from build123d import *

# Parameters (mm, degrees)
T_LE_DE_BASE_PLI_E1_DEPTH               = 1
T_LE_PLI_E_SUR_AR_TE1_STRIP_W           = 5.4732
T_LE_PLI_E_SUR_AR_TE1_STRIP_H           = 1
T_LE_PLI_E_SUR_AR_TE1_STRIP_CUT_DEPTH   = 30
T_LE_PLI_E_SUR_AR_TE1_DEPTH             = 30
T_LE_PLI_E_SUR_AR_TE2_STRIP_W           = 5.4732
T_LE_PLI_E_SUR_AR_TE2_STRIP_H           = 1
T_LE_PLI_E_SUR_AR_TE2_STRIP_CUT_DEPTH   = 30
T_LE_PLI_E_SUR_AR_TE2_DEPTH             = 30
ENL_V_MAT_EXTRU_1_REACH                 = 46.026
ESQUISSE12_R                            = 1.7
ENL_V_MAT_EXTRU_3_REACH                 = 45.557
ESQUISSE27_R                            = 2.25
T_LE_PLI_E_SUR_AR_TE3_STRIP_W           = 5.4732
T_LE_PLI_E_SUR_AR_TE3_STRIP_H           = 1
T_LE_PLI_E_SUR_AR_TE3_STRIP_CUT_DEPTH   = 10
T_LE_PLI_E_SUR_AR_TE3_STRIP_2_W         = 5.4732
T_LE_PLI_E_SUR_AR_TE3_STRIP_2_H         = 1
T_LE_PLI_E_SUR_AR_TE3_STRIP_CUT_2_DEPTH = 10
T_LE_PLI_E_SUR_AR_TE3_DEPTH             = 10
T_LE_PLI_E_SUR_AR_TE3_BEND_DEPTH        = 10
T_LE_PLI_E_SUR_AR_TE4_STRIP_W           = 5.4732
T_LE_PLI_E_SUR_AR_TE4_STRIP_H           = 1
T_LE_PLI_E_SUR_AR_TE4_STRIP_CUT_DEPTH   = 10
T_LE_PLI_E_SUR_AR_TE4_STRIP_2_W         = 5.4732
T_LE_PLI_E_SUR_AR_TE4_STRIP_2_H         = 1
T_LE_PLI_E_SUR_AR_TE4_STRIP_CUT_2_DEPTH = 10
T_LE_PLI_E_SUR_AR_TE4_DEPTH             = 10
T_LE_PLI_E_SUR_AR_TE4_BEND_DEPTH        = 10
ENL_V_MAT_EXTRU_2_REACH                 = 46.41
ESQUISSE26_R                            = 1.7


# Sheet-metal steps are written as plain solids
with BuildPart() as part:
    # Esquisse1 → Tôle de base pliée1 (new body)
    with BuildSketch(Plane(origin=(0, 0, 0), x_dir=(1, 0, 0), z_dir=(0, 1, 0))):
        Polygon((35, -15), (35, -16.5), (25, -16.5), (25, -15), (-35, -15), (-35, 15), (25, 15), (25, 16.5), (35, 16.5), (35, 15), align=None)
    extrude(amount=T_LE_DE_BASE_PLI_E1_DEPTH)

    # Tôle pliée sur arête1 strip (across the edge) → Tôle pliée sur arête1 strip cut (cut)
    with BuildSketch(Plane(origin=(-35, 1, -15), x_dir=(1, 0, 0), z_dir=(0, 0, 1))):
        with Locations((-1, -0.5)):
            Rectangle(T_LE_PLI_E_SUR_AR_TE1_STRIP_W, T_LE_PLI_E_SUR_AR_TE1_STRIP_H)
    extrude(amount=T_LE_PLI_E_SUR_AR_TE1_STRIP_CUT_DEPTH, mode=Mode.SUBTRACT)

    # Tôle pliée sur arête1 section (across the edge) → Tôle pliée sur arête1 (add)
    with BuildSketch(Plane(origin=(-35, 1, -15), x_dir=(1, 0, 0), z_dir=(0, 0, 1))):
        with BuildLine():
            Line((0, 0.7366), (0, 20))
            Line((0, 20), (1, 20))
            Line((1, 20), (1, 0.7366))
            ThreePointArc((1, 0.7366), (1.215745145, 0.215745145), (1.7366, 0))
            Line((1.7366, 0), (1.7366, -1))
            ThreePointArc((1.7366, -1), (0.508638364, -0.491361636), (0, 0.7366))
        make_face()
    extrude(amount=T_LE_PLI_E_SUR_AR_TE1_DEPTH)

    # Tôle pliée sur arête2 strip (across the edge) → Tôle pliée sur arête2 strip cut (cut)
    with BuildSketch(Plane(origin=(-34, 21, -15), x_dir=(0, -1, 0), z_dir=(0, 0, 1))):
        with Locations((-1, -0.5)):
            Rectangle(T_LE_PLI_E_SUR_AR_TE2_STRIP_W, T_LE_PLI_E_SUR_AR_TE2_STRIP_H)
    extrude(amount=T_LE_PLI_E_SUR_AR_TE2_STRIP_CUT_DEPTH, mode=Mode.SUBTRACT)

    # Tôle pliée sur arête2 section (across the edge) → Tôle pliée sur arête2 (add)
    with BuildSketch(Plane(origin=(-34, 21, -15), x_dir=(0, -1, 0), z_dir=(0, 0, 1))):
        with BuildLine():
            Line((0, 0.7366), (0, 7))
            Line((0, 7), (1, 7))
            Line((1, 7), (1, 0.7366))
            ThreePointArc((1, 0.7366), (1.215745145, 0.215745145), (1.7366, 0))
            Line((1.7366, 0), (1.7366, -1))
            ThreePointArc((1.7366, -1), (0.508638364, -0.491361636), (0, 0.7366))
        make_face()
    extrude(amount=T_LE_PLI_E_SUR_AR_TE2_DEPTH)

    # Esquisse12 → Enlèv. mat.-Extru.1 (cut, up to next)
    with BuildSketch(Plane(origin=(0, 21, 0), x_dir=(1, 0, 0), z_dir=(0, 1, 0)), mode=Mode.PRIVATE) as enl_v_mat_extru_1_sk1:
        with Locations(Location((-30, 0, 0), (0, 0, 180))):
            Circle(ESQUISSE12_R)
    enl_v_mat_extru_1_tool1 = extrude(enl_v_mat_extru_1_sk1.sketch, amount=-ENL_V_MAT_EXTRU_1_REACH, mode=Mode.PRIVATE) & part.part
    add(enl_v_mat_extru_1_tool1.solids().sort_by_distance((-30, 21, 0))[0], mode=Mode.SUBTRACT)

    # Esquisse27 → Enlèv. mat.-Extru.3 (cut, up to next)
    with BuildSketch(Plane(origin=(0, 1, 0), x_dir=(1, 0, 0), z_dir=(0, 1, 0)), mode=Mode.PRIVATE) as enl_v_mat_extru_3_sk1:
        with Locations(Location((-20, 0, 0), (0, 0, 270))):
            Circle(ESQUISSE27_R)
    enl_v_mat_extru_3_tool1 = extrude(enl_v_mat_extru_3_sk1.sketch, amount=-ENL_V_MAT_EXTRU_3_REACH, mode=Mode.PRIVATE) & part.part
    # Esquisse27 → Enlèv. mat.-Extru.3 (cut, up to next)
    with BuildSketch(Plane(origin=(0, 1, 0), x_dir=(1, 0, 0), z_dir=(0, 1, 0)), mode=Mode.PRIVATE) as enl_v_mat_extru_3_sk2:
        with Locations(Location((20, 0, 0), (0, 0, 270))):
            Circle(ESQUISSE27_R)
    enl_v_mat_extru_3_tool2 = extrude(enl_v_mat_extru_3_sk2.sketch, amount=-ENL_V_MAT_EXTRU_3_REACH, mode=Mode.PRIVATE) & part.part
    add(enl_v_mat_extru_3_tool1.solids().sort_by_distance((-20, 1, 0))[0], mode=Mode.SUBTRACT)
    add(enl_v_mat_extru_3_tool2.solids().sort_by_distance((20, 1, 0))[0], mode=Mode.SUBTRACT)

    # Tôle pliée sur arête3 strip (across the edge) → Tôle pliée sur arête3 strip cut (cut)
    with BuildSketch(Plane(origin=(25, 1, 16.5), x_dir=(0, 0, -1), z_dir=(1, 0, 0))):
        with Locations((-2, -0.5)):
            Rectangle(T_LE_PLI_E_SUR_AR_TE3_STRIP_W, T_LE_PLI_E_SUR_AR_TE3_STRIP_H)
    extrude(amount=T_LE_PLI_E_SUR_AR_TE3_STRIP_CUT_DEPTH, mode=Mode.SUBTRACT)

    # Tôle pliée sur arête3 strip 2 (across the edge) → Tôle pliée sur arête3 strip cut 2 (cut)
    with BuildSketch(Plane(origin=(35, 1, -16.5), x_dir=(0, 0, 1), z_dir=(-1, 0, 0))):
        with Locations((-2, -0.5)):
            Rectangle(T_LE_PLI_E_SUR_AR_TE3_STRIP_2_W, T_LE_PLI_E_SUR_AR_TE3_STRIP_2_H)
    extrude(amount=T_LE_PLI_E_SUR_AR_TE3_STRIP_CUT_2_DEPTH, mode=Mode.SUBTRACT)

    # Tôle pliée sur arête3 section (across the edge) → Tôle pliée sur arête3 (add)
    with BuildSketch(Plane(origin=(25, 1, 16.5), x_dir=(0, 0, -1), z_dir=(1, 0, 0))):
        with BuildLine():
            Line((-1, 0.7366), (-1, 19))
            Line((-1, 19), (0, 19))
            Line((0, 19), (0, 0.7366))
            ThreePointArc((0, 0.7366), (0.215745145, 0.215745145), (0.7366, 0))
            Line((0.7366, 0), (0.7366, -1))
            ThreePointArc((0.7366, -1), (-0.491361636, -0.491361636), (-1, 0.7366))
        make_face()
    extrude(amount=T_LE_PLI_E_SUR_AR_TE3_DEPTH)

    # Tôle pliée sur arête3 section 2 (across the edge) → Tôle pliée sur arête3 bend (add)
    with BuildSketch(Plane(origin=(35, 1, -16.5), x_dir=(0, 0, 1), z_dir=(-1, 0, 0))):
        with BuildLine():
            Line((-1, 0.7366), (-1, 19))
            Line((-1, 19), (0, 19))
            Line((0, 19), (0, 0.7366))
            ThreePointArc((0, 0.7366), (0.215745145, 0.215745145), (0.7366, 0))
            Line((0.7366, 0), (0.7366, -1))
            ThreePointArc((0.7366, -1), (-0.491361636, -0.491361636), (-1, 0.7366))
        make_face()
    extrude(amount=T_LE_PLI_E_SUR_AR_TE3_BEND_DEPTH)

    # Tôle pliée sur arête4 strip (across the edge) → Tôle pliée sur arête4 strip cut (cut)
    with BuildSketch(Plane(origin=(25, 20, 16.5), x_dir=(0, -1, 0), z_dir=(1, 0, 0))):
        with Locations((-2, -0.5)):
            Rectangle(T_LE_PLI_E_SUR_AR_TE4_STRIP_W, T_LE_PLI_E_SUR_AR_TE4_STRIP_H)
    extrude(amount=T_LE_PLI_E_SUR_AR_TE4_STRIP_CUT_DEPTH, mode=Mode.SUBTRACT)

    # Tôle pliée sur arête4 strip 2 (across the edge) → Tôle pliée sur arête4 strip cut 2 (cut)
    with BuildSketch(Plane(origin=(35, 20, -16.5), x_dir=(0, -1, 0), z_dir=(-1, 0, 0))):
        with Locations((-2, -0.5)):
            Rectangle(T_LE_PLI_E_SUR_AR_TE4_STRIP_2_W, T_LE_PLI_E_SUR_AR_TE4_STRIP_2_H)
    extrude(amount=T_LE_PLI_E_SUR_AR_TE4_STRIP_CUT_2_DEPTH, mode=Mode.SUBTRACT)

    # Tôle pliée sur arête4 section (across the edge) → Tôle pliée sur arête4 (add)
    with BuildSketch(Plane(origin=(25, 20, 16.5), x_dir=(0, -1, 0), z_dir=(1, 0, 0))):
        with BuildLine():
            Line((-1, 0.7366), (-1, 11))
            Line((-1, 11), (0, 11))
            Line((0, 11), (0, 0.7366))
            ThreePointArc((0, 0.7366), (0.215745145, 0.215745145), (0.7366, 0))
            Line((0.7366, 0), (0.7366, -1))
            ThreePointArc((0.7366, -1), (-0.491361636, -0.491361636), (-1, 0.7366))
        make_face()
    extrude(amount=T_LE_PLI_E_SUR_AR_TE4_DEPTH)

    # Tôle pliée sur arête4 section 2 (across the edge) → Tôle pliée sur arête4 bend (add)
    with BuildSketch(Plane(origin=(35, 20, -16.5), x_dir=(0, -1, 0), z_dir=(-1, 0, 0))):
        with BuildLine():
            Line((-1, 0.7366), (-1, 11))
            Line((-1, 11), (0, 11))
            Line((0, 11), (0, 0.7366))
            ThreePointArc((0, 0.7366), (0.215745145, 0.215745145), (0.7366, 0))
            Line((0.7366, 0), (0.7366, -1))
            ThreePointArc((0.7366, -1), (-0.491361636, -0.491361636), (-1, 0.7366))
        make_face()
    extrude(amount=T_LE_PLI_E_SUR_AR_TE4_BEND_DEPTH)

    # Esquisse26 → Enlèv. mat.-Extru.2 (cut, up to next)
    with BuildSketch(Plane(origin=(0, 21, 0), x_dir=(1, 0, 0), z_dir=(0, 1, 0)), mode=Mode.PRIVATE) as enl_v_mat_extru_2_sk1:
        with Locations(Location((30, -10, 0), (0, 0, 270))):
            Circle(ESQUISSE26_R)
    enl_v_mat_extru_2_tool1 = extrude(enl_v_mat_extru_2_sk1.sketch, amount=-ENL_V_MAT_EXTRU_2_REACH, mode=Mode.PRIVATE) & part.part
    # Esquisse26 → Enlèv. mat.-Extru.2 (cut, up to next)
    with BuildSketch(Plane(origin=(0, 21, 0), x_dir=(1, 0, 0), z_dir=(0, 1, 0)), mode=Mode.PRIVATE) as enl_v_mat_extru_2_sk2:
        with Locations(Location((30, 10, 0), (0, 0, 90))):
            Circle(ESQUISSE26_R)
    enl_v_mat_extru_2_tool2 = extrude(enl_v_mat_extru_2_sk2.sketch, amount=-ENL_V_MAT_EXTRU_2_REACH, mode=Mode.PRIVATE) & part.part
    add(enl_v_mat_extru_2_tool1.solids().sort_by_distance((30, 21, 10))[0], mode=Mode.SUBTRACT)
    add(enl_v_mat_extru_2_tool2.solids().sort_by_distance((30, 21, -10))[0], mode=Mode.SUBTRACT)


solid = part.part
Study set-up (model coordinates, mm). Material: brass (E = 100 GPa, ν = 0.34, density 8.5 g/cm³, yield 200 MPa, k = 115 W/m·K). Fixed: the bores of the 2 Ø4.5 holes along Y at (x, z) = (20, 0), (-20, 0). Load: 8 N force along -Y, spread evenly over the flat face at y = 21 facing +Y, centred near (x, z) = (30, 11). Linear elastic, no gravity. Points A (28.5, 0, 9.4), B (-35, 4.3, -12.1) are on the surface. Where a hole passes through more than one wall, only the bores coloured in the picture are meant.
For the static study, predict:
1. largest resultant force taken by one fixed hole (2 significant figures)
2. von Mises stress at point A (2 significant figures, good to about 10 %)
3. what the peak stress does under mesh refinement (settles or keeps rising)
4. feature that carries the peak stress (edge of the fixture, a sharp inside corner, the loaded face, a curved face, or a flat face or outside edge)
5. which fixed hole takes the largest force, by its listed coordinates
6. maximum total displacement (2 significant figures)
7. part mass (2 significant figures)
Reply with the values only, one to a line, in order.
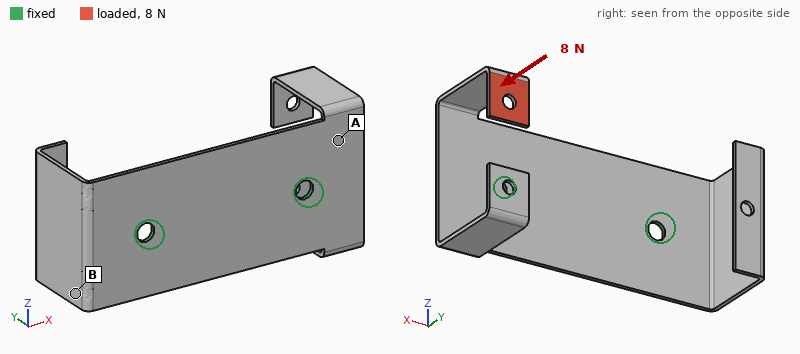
8.4 N
6.5 MPa
keeps rising
edge of the fixture
(20, 0)
0.23 mm
29 g
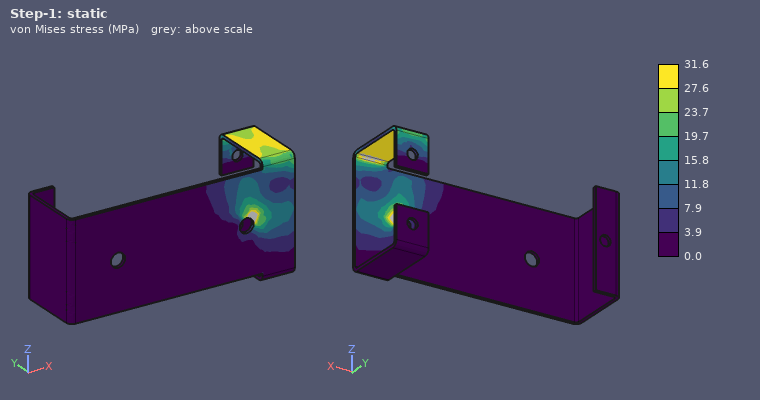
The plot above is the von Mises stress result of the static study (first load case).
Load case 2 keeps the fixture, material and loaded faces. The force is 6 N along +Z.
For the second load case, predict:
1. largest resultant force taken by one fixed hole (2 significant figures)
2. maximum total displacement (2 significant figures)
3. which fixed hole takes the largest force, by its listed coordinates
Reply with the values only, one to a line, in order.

7.2 N
0.54 mm
(20, 0)
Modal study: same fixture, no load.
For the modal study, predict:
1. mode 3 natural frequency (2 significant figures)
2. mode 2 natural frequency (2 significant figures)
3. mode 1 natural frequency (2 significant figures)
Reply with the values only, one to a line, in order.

480 Hz
470 Hz
450 Hz
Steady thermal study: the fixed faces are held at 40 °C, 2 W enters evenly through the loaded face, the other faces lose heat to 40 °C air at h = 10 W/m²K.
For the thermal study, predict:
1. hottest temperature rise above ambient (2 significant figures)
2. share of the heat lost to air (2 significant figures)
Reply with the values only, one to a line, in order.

61 K
17 %
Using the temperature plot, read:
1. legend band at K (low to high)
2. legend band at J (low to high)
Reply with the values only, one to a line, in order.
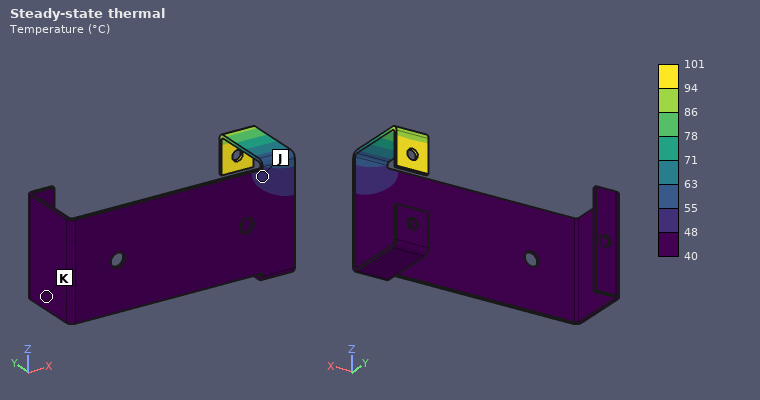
40 to 48 °C
48 to 55 °C
